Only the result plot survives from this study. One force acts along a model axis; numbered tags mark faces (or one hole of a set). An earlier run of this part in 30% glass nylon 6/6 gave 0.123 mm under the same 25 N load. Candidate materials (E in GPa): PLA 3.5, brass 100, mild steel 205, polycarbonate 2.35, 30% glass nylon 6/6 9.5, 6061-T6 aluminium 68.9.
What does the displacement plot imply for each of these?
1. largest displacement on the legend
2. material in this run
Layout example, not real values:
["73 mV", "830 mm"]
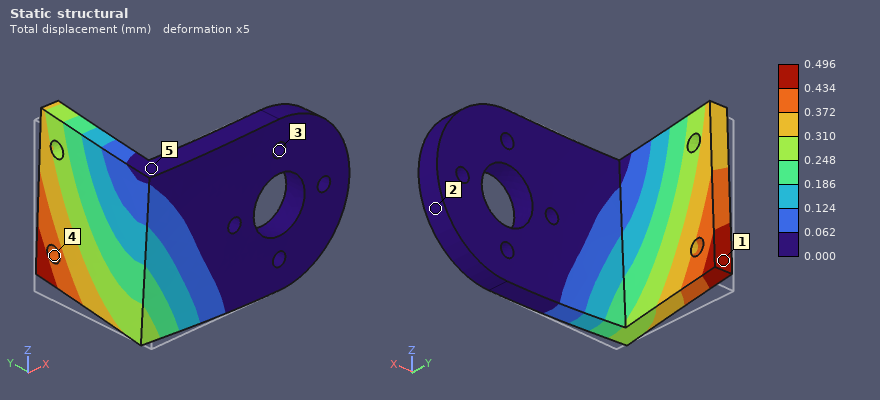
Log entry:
["0.496 mm", "polycarbonate"]
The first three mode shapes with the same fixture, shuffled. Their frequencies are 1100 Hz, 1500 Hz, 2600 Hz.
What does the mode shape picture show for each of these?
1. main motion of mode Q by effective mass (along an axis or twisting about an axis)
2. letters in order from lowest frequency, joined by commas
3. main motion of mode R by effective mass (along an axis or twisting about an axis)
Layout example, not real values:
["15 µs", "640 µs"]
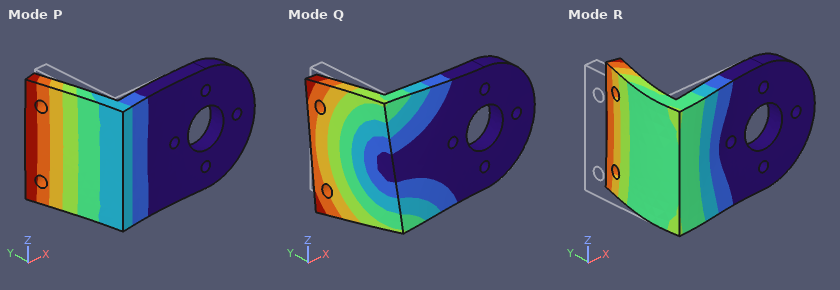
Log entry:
["along Z", "P, Q, R", "along Y"]
